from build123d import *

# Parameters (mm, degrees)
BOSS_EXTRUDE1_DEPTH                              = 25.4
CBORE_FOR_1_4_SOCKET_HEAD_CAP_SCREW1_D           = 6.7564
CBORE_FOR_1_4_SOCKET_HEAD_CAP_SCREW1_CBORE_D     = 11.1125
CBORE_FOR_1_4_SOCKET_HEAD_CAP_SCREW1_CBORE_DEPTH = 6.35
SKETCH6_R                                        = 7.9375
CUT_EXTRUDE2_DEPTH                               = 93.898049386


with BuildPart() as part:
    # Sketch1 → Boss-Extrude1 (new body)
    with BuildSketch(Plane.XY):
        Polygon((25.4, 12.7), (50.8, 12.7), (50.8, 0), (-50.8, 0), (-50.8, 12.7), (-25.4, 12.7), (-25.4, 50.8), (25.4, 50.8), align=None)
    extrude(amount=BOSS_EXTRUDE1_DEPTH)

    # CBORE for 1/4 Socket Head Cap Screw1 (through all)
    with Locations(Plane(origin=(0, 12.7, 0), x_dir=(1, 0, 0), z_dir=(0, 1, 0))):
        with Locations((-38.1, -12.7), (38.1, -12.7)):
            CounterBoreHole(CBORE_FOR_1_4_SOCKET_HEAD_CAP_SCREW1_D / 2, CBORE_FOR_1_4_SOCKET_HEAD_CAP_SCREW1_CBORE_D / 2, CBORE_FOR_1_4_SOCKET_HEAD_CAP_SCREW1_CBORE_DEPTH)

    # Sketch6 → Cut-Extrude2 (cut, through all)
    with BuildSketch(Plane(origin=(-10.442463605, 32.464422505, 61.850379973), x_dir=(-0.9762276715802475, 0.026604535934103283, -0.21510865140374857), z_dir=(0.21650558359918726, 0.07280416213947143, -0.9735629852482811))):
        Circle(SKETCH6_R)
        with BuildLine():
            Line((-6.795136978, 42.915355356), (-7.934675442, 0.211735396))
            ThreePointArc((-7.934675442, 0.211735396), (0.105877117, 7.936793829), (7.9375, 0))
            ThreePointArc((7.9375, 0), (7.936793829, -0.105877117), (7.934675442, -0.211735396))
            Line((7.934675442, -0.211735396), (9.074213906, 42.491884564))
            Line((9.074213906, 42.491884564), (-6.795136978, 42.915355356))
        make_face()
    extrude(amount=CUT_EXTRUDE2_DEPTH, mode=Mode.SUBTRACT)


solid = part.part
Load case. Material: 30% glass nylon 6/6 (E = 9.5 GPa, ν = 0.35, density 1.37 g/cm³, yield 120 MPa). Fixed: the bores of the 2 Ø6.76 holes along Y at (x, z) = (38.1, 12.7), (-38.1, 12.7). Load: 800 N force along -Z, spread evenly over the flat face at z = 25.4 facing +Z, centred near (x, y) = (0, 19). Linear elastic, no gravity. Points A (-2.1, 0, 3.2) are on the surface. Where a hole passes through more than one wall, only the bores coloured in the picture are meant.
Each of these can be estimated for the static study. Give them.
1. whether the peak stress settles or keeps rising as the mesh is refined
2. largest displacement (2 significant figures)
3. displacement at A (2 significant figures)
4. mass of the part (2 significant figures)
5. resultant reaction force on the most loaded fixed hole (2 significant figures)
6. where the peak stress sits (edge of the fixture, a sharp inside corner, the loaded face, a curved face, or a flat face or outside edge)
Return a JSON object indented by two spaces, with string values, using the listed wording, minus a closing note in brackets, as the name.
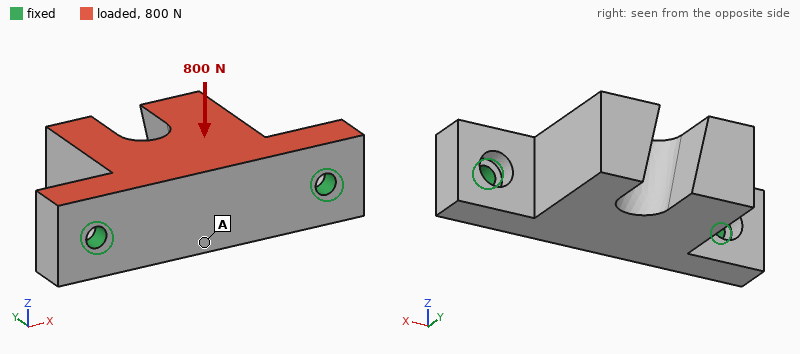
{
  "whether the peak stress settles or keeps rising as the mesh is refined": "keeps rising",
  "largest displacement": "0.23 mm",
  "displacement at A": "0.039 mm",
  "mass of the part": "98 g",
  "resultant reaction force on the most loaded fixed hole": "400 N",
  "where the peak stress sits": "edge of the fixture"
}
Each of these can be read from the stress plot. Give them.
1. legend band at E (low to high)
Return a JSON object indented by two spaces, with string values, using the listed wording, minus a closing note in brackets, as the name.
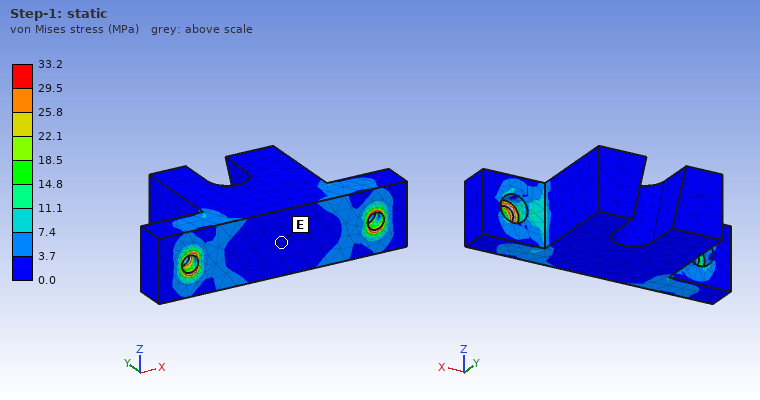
{
  "legend band at E": "0.0 to 3.7 MPa"
}
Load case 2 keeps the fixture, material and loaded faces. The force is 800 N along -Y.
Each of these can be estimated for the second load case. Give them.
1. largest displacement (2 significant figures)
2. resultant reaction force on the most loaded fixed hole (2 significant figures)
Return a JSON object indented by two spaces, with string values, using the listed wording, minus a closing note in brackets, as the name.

{
  "largest displacement": "0.16 mm",
  "resultant reaction force on the most loaded fixed hole": "470 N"
}
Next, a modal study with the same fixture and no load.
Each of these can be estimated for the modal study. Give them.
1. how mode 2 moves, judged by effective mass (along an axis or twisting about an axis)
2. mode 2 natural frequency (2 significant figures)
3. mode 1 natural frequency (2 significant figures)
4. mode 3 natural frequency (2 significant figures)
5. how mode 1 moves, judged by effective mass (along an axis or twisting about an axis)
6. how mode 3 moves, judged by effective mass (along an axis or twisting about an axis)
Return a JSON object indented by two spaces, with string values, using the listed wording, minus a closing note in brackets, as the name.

{
  "how mode 2 moves, judged by effective mass": "along Y",
  "mode 2 natural frequency": "3600 Hz",
  "mode 1 natural frequency": "1200 Hz",
  "mode 3 natural frequency": "4100 Hz",
  "how mode 1 moves, judged by effective mass": "along Z",
  "how mode 3 moves, judged by effective mass": "along X"
}
